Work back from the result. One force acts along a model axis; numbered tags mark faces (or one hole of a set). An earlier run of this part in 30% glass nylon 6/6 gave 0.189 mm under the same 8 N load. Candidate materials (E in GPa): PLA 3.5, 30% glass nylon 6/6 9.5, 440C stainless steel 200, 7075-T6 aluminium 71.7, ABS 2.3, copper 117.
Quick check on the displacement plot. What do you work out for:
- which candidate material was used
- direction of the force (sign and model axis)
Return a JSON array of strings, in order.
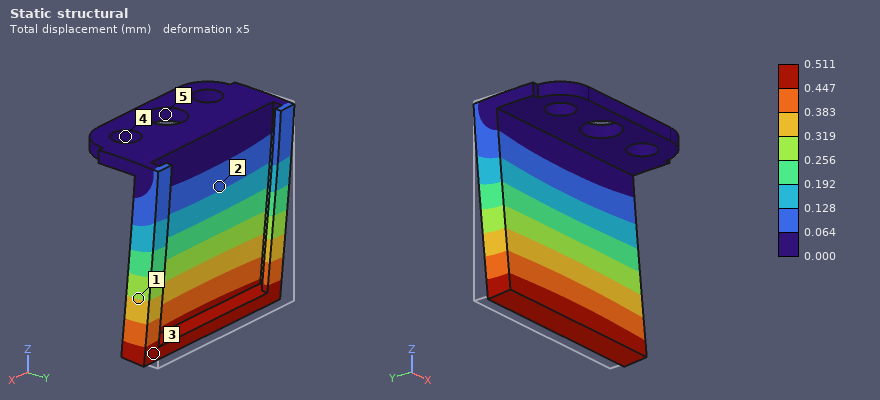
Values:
["PLA", "-Y"]
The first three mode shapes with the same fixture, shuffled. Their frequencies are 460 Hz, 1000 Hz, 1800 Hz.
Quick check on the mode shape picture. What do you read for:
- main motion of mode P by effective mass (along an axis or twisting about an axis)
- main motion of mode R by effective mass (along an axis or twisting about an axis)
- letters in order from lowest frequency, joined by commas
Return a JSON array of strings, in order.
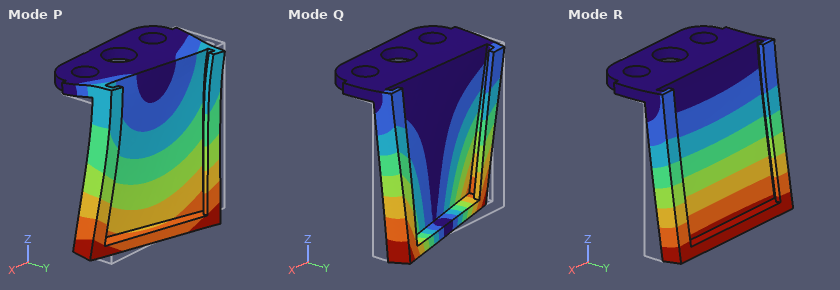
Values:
["along X", "along Y", "R, Q, P"]
